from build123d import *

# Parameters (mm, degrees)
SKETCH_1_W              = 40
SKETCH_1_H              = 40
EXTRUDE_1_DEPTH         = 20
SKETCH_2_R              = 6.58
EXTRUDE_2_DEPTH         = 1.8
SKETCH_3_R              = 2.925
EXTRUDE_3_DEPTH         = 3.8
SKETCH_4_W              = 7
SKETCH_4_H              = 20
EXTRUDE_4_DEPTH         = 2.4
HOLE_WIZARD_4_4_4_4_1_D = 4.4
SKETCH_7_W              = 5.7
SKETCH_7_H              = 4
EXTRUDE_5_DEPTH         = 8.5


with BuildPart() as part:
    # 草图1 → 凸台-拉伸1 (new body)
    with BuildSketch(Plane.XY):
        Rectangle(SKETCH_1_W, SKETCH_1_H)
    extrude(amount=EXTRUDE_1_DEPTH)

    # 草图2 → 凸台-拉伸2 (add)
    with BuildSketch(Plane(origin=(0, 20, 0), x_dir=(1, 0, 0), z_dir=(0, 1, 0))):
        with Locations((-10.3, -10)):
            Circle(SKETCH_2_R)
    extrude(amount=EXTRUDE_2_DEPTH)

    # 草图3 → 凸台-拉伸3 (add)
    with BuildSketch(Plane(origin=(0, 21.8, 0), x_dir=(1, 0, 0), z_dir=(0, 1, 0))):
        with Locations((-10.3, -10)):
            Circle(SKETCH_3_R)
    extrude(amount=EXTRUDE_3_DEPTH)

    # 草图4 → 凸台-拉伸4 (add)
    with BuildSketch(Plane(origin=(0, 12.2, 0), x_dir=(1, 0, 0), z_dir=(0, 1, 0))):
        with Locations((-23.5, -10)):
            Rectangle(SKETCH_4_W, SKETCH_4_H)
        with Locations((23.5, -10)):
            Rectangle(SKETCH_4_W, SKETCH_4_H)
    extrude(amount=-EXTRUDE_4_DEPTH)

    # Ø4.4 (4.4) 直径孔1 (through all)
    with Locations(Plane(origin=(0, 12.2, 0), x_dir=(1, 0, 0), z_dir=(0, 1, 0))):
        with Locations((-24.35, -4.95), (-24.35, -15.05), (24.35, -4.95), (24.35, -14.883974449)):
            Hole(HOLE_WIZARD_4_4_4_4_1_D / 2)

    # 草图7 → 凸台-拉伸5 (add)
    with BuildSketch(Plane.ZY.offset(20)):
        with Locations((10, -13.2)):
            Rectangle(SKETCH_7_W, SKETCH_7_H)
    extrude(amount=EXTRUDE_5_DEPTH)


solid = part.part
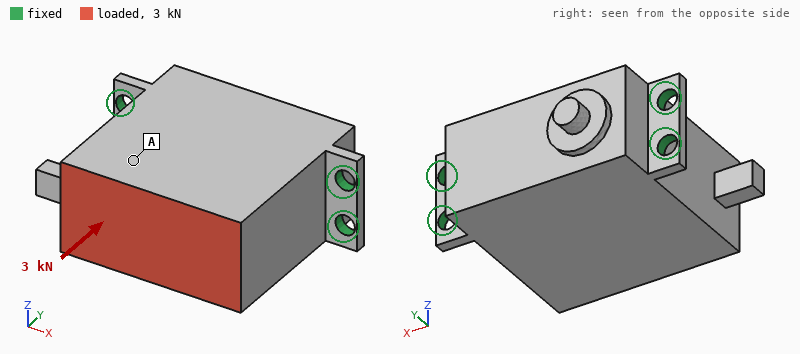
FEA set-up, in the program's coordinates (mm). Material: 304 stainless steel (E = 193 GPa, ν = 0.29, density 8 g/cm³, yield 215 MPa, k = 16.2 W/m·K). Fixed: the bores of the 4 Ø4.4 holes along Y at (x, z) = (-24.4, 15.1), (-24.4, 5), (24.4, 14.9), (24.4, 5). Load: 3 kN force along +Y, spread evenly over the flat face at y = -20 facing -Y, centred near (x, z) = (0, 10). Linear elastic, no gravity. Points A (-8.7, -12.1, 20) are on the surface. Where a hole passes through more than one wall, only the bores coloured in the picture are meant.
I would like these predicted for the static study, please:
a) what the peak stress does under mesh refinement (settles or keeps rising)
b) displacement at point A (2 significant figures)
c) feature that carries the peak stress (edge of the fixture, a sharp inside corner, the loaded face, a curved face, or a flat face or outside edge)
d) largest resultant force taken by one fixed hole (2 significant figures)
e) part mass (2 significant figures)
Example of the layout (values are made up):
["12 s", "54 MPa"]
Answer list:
["keeps rising", "4.1 µm", "edge of the fixture", "760 N", "260 g"]
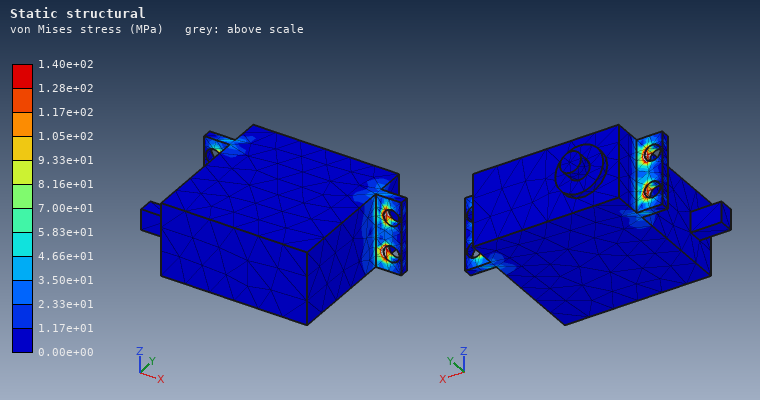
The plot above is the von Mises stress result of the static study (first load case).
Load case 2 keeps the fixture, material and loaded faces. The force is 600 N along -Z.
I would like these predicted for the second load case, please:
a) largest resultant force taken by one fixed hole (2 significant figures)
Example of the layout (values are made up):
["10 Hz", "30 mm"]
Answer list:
["770 N"]
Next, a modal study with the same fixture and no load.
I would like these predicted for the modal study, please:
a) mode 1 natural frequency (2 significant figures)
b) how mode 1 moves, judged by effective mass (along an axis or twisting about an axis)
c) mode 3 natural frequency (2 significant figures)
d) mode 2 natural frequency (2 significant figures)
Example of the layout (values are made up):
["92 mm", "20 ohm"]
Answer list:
["3000 Hz", "along Z", "8800 Hz", "8700 Hz"]
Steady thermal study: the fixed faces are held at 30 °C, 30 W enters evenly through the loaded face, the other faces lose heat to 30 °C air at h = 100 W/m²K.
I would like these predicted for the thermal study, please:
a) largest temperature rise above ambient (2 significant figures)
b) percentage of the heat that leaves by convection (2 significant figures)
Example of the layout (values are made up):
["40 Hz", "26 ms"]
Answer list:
["75 K", "74 %"]
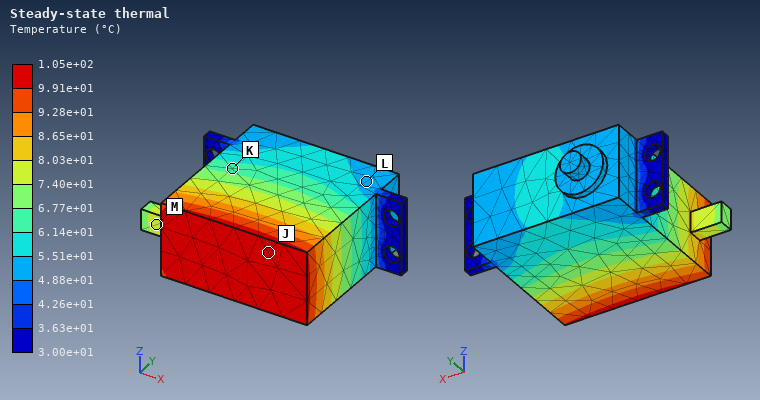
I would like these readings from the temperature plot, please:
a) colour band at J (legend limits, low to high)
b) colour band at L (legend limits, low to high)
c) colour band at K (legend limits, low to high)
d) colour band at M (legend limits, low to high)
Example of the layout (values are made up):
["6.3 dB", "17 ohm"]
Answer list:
["9.91e+01 to 1.05e+02 °C", "4.88e+01 to 5.51e+01 °C", "6.14e+01 to 6.77e+01 °C", "7.40e+01 to 8.03e+01 °C"]
